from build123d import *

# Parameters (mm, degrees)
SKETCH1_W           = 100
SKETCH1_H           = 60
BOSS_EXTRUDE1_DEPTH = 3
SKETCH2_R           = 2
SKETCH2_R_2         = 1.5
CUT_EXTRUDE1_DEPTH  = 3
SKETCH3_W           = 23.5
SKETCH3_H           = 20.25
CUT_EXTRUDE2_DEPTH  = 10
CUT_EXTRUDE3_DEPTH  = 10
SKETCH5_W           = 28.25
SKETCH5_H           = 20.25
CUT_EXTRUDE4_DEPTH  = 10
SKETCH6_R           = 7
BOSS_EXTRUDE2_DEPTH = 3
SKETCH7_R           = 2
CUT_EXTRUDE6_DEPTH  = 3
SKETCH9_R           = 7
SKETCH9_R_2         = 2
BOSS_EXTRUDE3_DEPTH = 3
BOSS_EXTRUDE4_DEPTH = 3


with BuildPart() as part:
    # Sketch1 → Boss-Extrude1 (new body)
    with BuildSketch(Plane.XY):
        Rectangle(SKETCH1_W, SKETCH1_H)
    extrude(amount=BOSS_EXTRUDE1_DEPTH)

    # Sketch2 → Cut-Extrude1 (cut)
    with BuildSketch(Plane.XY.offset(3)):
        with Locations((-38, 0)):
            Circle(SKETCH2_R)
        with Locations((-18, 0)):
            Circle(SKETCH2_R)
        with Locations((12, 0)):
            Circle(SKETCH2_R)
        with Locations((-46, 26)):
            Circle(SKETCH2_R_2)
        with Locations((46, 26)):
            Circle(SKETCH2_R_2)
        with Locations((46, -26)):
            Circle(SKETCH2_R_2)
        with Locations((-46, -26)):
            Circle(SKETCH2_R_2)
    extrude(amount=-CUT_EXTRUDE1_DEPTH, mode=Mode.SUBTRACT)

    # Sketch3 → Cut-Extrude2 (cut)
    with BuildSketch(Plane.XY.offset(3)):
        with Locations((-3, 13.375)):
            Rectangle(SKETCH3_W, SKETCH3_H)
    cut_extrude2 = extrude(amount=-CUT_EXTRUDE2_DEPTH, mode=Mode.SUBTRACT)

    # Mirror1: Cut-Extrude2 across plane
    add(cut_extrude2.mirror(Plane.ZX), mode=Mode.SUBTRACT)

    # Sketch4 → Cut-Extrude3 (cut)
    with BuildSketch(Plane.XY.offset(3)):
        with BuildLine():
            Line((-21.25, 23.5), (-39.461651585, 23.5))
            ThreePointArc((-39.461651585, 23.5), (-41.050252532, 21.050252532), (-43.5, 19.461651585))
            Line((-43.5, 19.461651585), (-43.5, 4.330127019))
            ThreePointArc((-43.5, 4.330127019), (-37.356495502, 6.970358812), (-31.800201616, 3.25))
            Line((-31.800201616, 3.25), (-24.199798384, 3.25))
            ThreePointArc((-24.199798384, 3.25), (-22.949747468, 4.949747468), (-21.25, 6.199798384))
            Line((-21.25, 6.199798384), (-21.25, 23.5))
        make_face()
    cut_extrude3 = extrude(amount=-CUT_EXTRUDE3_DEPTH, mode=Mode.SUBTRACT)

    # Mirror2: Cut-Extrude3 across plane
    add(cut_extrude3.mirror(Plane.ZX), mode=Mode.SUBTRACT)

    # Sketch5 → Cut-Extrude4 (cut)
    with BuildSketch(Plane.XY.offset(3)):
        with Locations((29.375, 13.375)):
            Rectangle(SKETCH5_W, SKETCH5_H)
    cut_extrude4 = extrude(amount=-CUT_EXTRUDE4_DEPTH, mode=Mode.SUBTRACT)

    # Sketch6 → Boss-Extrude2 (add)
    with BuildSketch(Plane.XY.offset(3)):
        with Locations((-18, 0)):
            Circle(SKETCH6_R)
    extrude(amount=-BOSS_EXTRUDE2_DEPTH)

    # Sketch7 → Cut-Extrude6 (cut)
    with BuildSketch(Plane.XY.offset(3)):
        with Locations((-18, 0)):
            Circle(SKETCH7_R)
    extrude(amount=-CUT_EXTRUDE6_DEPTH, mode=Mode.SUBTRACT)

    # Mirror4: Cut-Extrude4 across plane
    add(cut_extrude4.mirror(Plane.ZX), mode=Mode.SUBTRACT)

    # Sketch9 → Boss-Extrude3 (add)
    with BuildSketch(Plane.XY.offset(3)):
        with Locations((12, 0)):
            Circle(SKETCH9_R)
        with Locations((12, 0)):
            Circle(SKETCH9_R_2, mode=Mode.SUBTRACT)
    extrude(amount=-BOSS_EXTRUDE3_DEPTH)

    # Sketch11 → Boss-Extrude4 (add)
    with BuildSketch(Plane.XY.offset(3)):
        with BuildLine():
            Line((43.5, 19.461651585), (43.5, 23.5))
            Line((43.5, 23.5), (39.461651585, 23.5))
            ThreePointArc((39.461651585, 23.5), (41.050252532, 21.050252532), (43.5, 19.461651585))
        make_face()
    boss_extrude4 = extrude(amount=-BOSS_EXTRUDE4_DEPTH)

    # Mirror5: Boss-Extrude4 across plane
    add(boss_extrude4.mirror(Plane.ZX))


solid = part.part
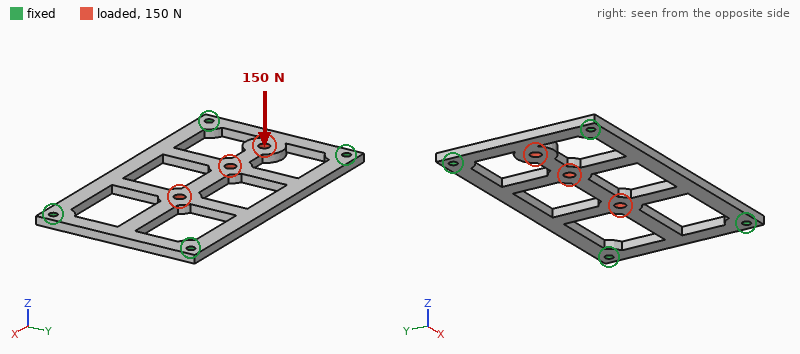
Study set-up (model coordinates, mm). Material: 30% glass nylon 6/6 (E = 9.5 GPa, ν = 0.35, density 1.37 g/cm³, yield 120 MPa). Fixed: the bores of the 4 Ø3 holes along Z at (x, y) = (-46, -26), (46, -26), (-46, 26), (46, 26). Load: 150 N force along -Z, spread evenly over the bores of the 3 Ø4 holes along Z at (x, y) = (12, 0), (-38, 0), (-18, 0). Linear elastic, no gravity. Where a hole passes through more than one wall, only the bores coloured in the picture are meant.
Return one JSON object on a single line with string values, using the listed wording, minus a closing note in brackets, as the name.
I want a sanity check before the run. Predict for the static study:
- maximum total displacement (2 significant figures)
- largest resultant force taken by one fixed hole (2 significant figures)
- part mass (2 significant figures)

{"maximum total displacement": "1.2 mm", "largest resultant force taken by one fixed hole": "51 N", "part mass": "13 g"}
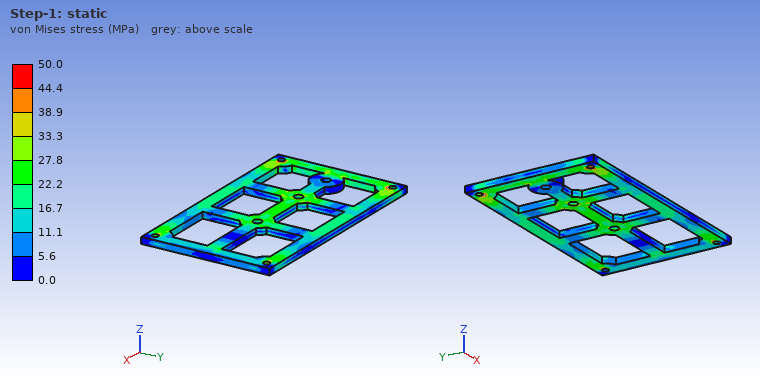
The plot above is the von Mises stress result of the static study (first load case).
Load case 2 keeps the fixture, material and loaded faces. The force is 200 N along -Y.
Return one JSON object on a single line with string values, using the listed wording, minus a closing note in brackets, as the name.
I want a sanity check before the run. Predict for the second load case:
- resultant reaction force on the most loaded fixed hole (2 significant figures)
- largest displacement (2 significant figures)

{"resultant reaction force on the most loaded fixed hole": "77 N", "largest displacement": "0.10 mm"}
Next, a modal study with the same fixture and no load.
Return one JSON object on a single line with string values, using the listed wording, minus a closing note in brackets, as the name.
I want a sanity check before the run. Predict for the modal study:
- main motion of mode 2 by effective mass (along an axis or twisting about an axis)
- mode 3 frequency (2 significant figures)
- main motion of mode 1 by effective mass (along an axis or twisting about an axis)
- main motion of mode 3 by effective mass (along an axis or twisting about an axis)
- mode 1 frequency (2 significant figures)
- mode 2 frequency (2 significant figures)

{"main motion of mode 2 by effective mass": "twisting about X", "mode 3 frequency": "1800 Hz", "main motion of mode 1 by effective mass": "along Z", "main motion of mode 3 by effective mass": "twisting about Y", "mode 1 frequency": "760 Hz", "mode 2 frequency": "1200 Hz"}
